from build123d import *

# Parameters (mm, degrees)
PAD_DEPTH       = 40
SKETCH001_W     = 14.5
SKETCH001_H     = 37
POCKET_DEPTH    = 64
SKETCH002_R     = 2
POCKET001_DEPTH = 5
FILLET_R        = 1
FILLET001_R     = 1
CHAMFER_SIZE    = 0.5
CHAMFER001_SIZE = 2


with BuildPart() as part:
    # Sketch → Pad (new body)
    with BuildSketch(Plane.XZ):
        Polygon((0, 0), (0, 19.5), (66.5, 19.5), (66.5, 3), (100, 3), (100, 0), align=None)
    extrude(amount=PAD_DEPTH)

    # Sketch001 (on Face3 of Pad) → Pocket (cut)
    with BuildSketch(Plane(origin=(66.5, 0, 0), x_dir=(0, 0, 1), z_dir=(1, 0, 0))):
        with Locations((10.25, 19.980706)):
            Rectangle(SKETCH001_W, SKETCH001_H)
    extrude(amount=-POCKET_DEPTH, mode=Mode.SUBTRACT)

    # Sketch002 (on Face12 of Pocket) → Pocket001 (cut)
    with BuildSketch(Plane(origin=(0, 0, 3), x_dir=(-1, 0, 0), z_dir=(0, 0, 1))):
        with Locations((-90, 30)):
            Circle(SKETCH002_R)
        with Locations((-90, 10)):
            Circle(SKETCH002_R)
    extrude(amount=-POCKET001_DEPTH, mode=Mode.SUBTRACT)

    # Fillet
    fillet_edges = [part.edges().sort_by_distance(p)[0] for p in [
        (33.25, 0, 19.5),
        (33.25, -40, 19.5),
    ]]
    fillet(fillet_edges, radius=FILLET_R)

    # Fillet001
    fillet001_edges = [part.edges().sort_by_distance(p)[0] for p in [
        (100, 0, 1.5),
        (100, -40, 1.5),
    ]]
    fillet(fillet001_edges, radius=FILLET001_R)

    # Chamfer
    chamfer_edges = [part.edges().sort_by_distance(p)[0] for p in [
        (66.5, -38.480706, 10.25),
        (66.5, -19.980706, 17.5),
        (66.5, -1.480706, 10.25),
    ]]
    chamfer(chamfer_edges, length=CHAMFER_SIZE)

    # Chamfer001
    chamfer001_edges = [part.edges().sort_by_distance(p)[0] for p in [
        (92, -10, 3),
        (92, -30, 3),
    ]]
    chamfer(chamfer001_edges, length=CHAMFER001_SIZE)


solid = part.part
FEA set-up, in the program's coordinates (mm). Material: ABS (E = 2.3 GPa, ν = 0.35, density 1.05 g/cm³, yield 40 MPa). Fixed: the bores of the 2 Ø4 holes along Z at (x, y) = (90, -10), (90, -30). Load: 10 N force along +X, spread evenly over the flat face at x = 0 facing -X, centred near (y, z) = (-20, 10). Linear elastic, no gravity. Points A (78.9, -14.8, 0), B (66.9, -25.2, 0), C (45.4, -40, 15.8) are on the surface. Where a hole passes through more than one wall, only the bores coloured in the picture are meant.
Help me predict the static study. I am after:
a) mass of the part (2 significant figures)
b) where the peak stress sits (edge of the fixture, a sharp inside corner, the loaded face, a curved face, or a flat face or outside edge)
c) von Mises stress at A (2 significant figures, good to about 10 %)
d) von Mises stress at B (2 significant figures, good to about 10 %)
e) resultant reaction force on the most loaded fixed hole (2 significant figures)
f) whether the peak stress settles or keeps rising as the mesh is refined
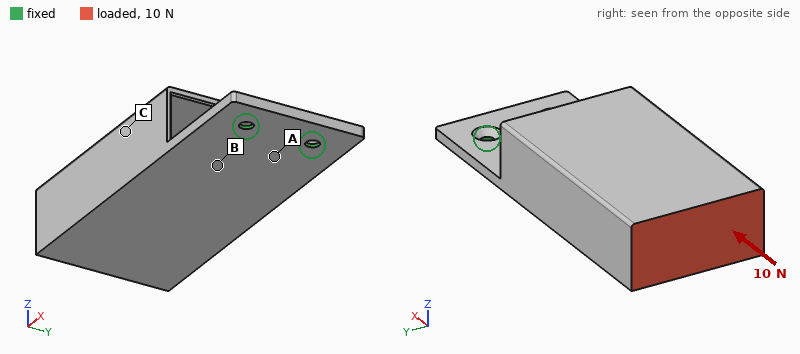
22 g
edge of the fixture
1.2 MPa
1.0 MPa
5.8 N
keeps rising
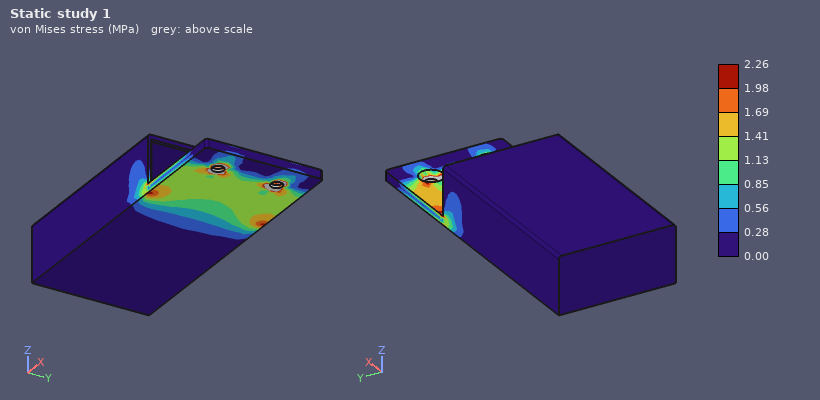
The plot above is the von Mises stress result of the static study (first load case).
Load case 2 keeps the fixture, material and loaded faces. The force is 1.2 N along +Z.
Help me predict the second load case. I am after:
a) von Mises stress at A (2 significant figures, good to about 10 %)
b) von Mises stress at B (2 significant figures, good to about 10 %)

1.5 MPa
1.1 MPa
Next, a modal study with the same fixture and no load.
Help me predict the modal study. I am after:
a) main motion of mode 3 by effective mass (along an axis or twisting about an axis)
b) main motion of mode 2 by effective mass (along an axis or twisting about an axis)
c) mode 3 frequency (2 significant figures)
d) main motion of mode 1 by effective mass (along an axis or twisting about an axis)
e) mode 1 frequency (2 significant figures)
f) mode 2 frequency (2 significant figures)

along Y
along Y
560 Hz
along Z
54 Hz
280 Hz
